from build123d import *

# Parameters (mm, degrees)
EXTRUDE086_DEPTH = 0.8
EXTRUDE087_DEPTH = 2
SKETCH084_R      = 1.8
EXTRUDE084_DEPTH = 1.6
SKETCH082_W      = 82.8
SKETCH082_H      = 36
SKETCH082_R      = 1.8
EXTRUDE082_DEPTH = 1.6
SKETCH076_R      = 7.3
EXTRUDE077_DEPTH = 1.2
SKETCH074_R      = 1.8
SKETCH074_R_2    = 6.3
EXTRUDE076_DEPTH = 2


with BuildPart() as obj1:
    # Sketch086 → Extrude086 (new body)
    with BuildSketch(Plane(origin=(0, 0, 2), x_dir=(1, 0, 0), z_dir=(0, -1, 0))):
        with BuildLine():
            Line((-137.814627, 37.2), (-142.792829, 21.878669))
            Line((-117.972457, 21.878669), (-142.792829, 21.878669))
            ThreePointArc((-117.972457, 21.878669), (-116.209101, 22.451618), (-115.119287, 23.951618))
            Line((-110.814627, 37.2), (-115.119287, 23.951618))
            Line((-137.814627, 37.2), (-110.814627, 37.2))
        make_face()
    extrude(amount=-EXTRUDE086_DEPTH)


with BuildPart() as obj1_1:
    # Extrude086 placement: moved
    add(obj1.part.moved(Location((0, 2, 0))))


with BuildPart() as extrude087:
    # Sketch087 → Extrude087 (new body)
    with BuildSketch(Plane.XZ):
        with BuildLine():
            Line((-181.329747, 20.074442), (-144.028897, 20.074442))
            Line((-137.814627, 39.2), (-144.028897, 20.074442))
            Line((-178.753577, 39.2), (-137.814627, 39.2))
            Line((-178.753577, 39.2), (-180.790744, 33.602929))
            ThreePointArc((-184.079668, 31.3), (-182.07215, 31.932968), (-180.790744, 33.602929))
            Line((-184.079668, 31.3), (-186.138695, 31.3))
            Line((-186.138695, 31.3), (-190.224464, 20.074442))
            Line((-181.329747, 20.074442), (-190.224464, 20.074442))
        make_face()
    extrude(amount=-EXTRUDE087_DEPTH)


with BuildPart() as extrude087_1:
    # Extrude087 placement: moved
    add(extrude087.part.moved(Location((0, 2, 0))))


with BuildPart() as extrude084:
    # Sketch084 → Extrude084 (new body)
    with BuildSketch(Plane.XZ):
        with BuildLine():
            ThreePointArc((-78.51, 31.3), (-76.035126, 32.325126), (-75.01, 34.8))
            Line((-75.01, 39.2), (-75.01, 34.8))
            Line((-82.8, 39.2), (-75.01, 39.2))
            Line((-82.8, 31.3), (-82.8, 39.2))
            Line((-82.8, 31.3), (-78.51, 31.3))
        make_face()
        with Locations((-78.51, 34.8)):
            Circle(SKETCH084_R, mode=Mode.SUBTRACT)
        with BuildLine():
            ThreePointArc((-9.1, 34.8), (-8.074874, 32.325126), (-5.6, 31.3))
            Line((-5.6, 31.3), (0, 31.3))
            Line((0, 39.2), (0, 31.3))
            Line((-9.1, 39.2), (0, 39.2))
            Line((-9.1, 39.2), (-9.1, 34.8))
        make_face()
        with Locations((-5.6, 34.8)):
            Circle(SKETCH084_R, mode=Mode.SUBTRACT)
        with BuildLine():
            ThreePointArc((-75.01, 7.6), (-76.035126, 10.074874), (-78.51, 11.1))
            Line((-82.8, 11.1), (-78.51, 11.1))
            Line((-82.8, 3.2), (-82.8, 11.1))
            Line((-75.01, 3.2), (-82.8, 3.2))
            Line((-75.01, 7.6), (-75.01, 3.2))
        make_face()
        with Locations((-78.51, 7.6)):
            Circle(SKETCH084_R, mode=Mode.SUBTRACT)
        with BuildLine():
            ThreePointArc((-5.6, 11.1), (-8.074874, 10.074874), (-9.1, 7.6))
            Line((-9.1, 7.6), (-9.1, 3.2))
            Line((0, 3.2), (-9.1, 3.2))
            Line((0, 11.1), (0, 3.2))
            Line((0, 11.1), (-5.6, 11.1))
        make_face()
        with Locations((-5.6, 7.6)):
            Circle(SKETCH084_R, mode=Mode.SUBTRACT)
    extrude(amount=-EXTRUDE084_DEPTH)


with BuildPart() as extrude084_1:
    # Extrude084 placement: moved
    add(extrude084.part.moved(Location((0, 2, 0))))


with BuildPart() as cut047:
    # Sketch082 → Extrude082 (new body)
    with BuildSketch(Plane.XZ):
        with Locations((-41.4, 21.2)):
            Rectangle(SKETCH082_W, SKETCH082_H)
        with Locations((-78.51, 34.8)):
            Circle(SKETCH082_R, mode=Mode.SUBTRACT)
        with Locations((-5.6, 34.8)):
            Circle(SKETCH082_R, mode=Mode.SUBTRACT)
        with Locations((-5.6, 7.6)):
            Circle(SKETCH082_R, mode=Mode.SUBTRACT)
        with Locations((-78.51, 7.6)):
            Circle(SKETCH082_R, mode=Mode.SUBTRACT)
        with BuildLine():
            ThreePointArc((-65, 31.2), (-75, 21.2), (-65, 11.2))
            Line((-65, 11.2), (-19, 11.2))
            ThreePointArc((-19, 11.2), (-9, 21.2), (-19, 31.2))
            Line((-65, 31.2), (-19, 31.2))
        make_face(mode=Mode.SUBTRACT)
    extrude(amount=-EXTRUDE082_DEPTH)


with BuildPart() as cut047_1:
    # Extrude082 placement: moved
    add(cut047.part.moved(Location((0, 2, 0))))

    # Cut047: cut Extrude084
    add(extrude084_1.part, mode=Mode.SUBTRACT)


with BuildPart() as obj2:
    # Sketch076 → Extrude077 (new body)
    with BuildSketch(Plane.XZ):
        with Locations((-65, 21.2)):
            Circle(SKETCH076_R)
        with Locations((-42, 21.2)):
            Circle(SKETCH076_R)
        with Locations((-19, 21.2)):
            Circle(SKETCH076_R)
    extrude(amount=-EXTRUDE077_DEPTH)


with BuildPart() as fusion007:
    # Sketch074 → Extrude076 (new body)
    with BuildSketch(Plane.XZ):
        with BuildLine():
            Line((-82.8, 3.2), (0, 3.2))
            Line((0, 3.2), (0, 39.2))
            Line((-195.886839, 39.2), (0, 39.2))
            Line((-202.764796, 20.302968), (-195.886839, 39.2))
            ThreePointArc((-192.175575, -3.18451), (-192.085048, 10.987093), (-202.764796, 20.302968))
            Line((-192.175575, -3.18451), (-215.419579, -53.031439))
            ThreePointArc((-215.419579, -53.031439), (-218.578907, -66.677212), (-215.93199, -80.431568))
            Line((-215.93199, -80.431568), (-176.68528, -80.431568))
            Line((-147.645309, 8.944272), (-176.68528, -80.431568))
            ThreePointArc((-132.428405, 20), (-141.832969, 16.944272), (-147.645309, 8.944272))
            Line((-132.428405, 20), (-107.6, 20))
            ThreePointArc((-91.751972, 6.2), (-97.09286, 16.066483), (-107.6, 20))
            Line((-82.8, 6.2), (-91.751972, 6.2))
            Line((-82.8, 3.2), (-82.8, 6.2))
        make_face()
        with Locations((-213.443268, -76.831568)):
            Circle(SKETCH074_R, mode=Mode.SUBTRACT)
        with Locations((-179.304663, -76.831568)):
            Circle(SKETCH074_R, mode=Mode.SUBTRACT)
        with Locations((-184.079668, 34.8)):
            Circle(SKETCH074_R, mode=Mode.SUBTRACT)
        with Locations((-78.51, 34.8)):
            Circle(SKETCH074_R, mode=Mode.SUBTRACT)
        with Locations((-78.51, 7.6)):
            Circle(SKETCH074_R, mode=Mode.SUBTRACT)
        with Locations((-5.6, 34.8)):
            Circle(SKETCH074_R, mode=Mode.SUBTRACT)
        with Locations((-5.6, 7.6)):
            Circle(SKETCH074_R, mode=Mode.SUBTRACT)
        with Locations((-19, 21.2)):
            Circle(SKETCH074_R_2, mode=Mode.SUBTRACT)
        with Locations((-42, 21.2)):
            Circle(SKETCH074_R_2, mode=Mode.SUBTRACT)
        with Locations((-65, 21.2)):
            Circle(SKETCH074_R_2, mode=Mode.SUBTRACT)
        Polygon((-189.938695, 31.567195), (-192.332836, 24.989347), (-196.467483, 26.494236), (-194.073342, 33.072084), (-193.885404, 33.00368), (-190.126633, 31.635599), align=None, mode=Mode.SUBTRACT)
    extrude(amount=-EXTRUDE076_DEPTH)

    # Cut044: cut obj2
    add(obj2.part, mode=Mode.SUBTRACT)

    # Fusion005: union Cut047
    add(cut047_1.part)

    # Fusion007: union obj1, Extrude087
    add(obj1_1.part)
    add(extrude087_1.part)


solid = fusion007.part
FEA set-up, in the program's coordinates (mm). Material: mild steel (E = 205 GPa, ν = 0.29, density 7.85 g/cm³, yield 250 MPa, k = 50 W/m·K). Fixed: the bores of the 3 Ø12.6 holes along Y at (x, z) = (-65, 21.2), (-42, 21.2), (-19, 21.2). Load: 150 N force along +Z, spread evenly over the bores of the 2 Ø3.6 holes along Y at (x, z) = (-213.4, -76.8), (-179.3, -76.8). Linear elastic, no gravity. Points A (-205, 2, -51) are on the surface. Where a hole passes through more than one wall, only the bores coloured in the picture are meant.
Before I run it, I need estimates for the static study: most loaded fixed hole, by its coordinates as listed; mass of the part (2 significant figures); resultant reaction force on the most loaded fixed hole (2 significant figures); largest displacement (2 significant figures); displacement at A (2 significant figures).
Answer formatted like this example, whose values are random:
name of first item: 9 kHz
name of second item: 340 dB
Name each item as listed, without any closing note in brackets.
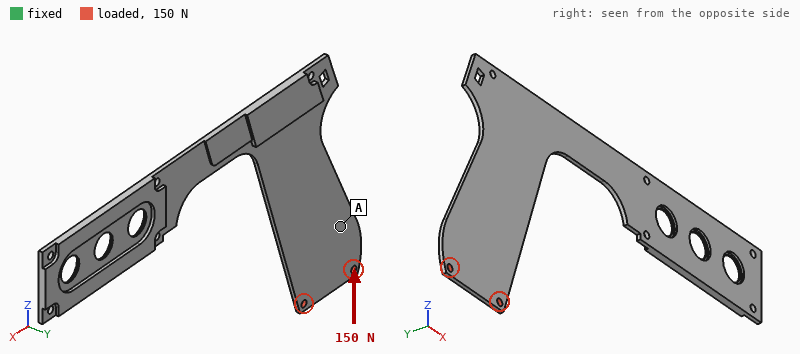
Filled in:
most loaded fixed hole, by its coordinates as listed: (-65, 21.2)
mass of the part: 180 g
resultant reaction force on the most loaded fixed hole: 490 N
largest displacement: 0.47 mm
displacement at A: 0.38 mm
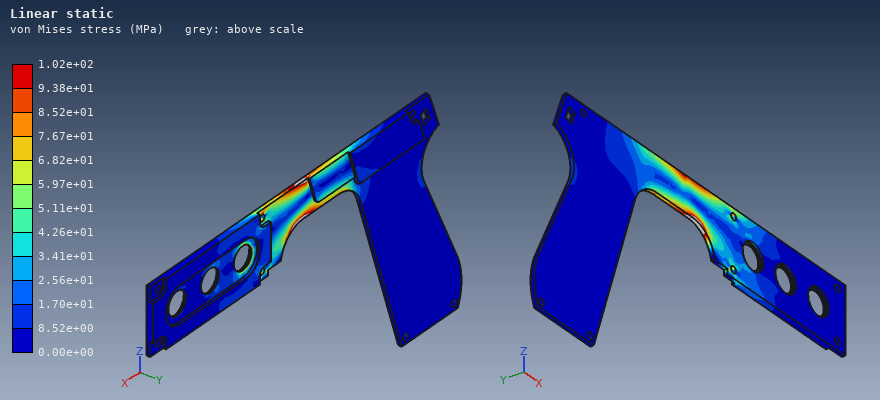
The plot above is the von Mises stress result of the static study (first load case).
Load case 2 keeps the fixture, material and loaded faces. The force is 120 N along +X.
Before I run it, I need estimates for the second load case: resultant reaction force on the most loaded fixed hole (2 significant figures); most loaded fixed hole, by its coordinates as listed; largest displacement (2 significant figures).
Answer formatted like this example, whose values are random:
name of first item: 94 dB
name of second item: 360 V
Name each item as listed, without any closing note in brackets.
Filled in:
resultant reaction force on the most loaded fixed hole: 240 N
most loaded fixed hole, by its coordinates as listed: (-65, 21.2)
largest displacement: 0.49 mm
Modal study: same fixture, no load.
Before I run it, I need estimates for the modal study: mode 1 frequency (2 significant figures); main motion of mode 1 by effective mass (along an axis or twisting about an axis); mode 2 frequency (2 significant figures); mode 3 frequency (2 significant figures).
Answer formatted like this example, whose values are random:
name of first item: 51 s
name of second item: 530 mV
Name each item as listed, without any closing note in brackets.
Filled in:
mode 1 frequency: 46 Hz
main motion of mode 1 by effective mass: along Y
mode 2 frequency: 140 Hz
mode 3 frequency: 380 Hz
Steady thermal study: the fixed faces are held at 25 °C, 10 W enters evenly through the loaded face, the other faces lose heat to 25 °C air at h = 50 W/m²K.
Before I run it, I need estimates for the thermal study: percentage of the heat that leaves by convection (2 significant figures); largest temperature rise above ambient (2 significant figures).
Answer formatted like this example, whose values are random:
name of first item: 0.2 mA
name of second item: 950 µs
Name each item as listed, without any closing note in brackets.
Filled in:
percentage of the heat that leaves by convection: 100 %
largest temperature rise above ambient: 87 K
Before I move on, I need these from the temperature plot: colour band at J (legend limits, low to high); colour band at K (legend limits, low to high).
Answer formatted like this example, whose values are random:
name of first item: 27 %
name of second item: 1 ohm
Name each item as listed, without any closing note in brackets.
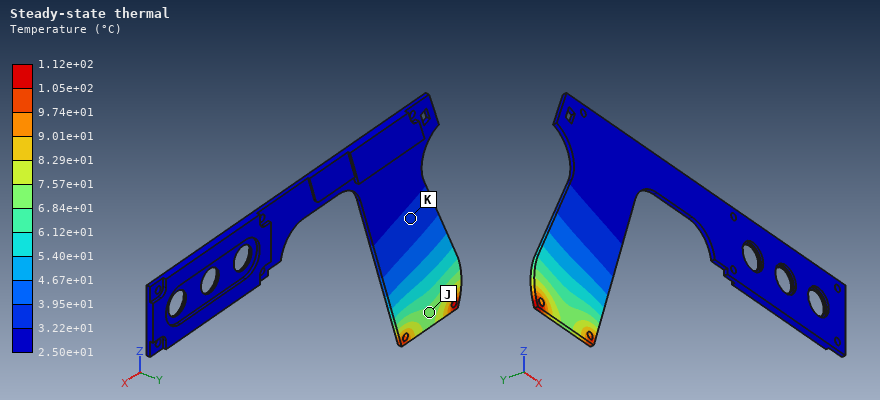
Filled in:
colour band at J: 6.84e+01 to 7.57e+01 °C
colour band at K: 3.22e+01 to 3.95e+01 °C
